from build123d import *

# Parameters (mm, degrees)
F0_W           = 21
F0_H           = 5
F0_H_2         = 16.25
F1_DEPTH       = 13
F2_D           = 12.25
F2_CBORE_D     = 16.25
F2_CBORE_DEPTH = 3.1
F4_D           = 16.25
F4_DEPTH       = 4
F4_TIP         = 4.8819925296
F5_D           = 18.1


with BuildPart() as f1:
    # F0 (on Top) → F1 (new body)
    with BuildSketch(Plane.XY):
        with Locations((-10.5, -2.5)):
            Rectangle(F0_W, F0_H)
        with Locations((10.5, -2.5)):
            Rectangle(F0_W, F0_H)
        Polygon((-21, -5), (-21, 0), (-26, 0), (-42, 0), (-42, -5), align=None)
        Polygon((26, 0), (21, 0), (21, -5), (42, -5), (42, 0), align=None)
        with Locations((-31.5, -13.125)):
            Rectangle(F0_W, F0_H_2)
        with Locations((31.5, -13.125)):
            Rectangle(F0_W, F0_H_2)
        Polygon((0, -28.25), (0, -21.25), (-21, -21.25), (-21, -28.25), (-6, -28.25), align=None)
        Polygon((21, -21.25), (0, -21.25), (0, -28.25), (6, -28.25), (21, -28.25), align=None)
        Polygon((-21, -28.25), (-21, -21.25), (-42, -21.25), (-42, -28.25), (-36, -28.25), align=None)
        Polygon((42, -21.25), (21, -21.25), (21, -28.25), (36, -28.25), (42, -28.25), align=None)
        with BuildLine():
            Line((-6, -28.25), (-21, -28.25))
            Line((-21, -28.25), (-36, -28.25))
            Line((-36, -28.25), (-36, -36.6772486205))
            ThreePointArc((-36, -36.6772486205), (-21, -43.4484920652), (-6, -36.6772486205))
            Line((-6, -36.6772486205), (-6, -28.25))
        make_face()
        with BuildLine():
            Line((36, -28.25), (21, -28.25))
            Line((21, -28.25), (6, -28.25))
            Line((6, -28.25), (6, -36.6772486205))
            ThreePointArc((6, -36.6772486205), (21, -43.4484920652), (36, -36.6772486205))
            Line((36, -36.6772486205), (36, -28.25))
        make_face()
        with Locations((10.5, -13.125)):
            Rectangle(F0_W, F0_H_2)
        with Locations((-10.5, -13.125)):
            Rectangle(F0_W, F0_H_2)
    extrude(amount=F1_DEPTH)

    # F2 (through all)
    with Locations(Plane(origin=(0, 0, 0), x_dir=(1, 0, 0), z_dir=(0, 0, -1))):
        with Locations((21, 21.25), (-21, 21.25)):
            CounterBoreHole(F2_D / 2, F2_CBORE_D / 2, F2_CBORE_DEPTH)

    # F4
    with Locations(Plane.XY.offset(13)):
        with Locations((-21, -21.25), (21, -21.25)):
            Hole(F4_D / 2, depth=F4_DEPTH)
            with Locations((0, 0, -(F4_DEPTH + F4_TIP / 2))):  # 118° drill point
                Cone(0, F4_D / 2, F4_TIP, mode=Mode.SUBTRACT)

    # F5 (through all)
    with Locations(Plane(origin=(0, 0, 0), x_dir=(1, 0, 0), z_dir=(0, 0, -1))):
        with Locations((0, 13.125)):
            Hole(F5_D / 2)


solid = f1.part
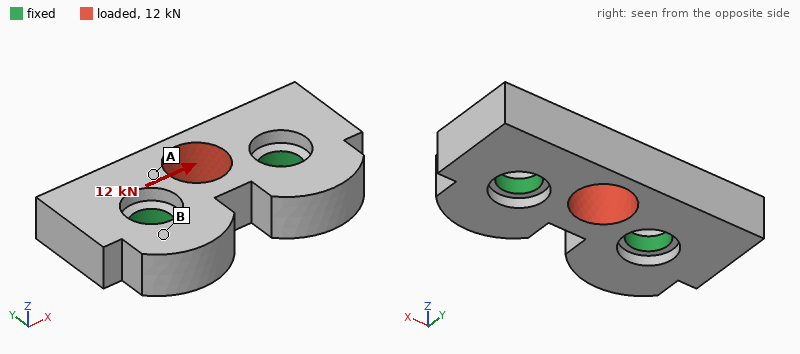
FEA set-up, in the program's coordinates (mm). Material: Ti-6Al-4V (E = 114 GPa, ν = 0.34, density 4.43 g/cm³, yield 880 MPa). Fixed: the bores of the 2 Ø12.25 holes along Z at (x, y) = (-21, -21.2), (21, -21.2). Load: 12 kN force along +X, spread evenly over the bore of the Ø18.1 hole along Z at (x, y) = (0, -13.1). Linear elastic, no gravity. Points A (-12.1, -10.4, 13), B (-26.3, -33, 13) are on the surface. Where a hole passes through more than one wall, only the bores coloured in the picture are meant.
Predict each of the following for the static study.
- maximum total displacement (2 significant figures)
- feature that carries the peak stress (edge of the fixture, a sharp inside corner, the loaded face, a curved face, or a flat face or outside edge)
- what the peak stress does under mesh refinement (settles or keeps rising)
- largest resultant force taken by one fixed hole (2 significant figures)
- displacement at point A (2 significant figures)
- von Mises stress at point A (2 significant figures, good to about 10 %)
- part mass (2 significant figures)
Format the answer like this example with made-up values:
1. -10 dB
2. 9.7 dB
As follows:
1. 9.8 µm
2. edge of the fixture
3. keeps rising
4. 6.1 kN
5. 6.1 µm
6. 26 MPa
7. 150 g
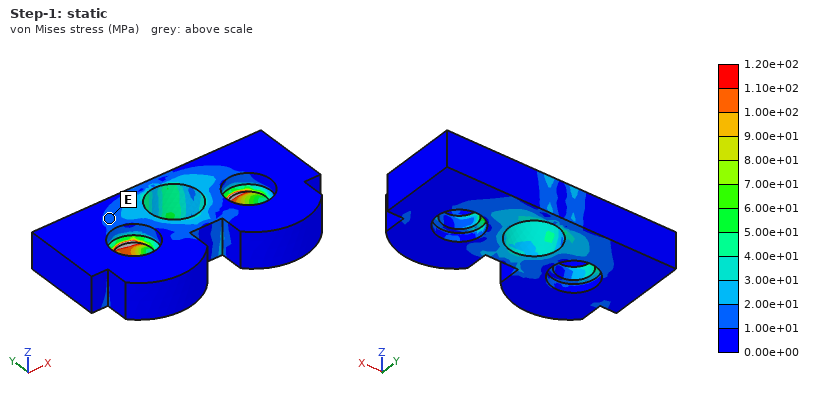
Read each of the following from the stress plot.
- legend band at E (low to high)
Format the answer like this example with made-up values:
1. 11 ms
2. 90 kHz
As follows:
1. 1.00e+01 to 2.00e+01 MPa
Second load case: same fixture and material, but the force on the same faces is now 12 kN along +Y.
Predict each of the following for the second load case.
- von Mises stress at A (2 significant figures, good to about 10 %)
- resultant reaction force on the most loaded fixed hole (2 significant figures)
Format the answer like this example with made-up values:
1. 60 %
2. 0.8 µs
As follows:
1. 26 MPa
2. 6.3 kN
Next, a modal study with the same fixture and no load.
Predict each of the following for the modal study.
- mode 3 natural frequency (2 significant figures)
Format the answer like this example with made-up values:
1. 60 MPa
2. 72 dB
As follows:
1. 13 kHz
